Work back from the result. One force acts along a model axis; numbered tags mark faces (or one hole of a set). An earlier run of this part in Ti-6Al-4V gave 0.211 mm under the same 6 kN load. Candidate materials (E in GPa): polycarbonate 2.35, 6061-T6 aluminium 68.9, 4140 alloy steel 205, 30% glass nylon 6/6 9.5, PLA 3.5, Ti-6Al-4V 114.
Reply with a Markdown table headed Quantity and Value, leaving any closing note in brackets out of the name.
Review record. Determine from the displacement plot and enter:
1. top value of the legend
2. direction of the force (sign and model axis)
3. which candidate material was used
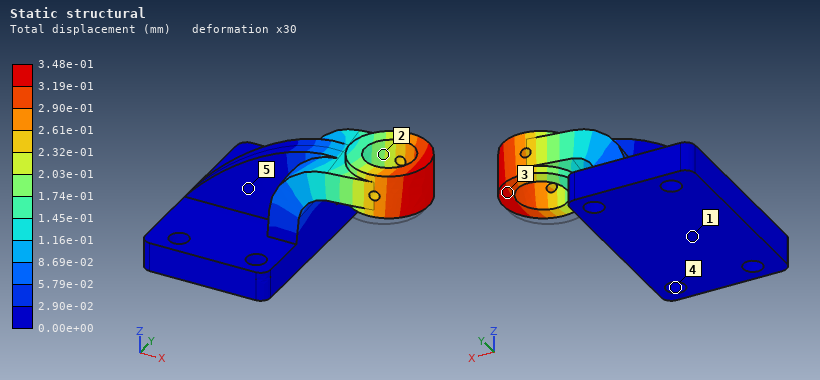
| Quantity | Value |
|---|---|
| top value of the legend | 3.48e-01 mm |
| direction of the force | +Y |
| which candidate material was used | 6061-T6 aluminium |
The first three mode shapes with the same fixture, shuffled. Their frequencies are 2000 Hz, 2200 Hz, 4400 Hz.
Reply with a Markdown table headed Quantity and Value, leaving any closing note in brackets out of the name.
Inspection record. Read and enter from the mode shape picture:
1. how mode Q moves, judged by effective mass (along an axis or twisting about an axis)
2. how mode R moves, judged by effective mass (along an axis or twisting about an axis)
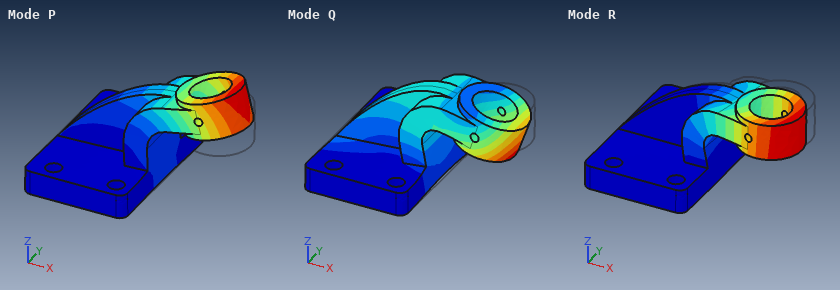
| Quantity | Value |
|---|---|
| how mode Q moves, judged by effective mass | along X |
| how mode R moves, judged by effective mass | along Y |
